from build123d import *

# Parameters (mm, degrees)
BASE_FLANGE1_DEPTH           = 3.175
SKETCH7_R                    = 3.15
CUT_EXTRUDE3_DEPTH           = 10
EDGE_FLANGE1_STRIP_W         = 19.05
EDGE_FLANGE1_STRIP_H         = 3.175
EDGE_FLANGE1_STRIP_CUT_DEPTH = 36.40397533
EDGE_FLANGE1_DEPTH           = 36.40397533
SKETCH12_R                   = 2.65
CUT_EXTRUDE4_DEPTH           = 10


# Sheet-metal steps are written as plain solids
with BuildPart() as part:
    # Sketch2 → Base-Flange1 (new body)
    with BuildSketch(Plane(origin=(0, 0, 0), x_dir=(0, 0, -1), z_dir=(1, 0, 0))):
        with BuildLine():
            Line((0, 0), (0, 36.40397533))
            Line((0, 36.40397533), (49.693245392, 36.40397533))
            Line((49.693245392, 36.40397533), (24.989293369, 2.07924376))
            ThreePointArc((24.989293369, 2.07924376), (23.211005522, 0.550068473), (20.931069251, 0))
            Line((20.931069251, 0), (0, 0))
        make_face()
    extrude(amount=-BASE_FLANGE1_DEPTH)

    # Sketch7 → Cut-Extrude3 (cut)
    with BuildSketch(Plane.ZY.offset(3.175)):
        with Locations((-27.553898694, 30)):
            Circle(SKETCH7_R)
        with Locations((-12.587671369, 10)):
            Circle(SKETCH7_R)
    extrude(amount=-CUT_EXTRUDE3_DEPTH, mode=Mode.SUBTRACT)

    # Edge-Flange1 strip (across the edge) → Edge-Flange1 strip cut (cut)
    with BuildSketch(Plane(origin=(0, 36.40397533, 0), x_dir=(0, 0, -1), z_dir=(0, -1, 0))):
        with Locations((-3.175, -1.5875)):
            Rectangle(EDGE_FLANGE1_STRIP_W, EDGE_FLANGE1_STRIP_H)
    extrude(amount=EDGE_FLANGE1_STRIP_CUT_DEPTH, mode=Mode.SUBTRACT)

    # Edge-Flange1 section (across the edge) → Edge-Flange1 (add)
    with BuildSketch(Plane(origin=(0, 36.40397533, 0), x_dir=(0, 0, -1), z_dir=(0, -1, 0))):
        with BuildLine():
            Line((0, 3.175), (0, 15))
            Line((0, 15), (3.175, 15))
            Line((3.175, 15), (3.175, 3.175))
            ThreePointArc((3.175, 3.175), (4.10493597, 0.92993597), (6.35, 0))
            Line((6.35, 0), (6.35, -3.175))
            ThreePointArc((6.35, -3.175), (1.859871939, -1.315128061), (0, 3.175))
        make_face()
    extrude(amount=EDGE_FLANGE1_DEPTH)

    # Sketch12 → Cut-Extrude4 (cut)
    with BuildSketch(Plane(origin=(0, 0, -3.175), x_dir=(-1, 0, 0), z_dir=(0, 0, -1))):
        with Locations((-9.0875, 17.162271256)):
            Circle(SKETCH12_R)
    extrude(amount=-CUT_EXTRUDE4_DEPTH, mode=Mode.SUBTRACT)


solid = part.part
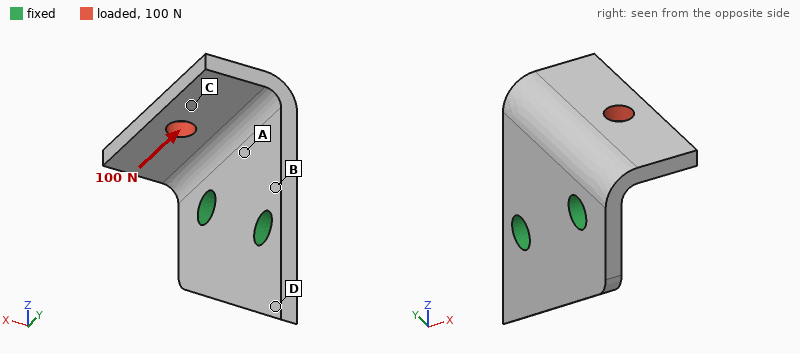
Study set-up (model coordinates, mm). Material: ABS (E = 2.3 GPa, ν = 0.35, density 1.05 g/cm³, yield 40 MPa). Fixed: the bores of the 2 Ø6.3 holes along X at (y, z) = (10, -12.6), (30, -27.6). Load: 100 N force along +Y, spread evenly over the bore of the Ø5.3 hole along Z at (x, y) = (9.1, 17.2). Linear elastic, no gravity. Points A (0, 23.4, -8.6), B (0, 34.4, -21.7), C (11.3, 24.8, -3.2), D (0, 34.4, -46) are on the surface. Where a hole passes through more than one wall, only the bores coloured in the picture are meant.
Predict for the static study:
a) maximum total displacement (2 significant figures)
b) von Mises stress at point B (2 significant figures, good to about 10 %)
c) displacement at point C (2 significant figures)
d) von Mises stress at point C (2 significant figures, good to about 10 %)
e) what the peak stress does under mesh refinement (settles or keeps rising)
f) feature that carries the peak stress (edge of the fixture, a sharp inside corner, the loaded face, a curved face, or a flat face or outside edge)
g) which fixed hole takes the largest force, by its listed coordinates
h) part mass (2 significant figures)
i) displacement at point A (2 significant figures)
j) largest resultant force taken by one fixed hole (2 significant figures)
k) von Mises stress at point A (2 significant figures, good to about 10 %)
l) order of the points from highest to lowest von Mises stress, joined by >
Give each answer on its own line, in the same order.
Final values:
0.76 mm
7.6 MPa
0.45 mm
3.1 MPa
keeps rising
edge of the fixture
(10, -12.6)
5.7 g
0.16 mm
110 N
6.0 MPa
B > A > C > D
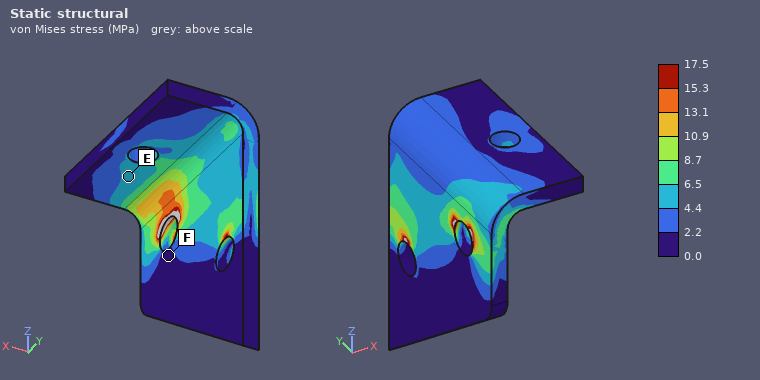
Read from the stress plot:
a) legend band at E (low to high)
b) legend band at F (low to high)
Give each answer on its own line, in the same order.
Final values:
4.4 to 6.5 MPa
0.0 to 2.2 MPa
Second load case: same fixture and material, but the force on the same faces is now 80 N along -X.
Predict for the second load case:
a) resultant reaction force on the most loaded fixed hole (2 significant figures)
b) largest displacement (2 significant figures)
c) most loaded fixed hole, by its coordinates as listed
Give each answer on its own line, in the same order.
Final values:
77 N
0.67 mm
(10, -12.6)
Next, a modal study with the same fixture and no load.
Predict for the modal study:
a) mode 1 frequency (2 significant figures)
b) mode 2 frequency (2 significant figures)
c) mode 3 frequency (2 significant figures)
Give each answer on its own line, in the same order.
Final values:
1200 Hz
1800 Hz
3000 Hz
